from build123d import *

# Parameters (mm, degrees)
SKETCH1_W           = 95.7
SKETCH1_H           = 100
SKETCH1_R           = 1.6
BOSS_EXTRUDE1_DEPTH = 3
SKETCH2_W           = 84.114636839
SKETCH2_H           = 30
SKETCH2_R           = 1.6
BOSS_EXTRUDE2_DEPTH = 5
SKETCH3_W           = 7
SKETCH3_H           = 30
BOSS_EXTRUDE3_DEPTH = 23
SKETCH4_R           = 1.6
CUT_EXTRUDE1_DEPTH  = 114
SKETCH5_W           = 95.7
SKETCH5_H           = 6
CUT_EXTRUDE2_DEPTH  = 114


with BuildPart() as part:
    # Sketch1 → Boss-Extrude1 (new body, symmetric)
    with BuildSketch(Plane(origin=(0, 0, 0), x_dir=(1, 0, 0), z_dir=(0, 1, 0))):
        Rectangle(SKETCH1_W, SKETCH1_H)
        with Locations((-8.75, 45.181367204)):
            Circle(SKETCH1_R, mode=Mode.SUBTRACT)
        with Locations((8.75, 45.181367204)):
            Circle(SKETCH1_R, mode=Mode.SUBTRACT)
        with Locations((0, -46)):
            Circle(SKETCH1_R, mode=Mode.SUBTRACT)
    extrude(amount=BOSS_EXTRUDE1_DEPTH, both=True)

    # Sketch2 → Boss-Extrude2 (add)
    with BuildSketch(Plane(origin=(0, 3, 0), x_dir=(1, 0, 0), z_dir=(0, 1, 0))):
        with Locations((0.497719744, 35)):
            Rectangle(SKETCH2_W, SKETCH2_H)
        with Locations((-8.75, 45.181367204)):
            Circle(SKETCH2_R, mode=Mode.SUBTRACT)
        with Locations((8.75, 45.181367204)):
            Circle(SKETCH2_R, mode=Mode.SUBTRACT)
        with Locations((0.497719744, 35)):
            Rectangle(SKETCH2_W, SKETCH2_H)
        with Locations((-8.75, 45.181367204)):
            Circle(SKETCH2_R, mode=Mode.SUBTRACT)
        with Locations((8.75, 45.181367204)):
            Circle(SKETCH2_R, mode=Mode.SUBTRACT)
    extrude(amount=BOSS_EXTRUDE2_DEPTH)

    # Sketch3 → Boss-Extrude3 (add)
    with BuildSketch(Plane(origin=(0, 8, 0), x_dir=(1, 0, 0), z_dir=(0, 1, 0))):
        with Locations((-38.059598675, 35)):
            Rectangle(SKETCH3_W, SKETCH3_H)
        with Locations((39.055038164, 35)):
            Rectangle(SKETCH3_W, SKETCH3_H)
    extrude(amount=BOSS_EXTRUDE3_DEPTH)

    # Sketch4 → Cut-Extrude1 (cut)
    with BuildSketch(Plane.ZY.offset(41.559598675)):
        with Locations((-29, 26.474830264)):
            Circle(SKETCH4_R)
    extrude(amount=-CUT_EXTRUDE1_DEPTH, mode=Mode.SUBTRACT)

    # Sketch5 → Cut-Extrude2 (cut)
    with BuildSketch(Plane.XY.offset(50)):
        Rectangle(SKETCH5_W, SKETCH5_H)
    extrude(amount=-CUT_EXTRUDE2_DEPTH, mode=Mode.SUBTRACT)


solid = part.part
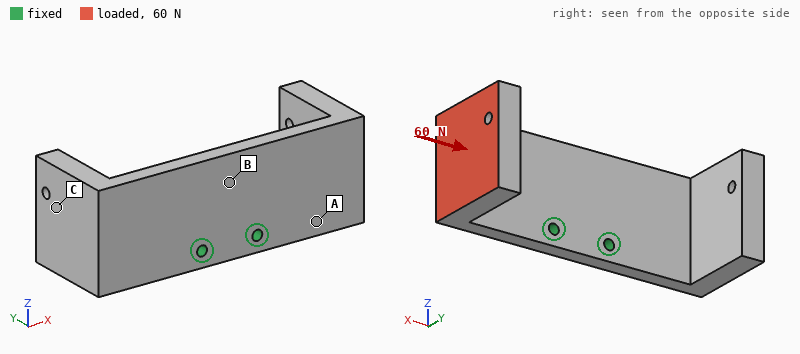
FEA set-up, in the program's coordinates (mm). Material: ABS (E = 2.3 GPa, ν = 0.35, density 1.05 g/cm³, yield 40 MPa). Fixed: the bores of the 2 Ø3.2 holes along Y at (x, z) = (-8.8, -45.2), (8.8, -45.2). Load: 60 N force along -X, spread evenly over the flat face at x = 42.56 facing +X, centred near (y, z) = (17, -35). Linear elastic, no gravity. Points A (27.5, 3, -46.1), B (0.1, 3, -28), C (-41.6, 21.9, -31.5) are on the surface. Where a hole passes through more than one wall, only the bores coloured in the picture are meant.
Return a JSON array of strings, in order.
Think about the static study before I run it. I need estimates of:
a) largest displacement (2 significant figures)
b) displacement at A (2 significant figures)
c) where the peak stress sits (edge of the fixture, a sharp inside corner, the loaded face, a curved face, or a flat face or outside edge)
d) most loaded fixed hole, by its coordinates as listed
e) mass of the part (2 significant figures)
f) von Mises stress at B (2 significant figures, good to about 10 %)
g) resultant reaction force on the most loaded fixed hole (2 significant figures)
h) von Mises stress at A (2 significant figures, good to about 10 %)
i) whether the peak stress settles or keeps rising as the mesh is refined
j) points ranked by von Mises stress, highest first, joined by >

["1.1 mm", "0.21 mm", "edge of the fixture", "(8.8, -45.2)", "23 g", "1.5 MPa", "54 N", "5.2 MPa", "keeps rising", "A > B > C"]
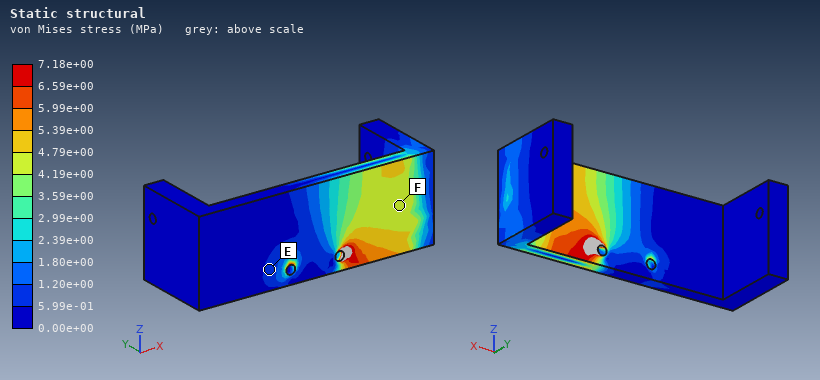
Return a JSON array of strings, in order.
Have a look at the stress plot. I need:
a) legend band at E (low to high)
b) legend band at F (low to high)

["5.99e-01 to 1.20e+00 MPa", "4.19e+00 to 4.79e+00 MPa"]
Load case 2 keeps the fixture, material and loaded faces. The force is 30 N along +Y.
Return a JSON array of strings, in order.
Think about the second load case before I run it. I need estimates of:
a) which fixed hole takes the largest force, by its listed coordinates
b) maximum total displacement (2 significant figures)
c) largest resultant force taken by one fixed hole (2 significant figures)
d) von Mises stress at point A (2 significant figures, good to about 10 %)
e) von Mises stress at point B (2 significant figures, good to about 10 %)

["(8.8, -45.2)", "1.1 mm", "57 N", "3.9 MPa", "2.9 MPa"]
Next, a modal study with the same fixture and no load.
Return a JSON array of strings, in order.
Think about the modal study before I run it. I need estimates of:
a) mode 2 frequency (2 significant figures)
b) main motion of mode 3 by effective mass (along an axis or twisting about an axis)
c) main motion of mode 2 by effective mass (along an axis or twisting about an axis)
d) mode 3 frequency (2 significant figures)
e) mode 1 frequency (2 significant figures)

["400 Hz", "along Z", "along Y", "620 Hz", "370 Hz"]
